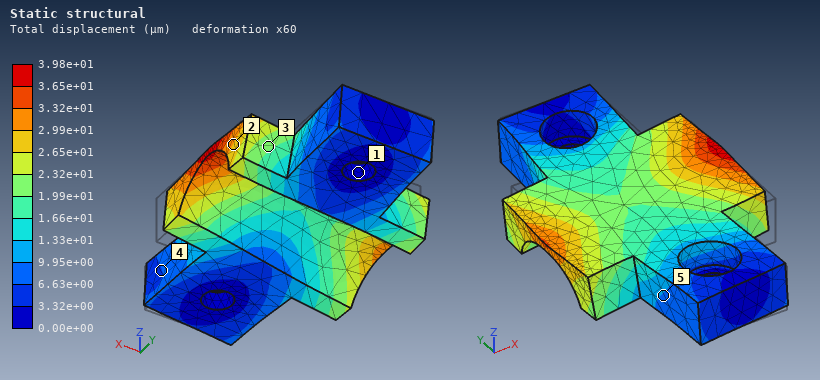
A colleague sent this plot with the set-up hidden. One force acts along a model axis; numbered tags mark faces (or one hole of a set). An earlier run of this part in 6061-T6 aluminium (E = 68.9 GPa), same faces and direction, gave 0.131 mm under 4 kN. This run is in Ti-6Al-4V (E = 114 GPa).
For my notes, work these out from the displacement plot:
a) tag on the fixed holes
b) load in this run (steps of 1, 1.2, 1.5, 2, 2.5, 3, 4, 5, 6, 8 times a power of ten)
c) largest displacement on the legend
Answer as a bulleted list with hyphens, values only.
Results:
- 1
- 2 kN
- 3.98e+01 µm
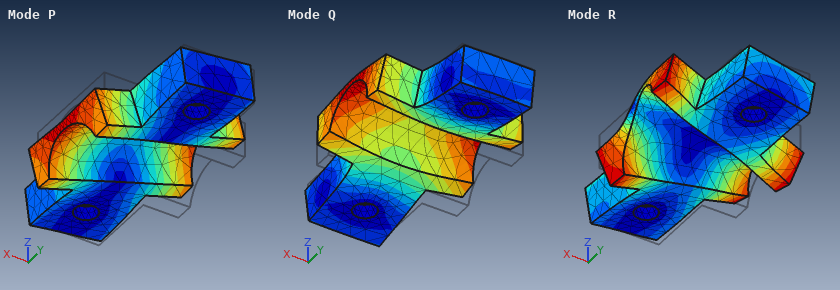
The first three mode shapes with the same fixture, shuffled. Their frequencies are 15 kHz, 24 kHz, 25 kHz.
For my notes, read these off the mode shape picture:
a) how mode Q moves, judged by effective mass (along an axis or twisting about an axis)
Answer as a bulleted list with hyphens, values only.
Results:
- along Z
